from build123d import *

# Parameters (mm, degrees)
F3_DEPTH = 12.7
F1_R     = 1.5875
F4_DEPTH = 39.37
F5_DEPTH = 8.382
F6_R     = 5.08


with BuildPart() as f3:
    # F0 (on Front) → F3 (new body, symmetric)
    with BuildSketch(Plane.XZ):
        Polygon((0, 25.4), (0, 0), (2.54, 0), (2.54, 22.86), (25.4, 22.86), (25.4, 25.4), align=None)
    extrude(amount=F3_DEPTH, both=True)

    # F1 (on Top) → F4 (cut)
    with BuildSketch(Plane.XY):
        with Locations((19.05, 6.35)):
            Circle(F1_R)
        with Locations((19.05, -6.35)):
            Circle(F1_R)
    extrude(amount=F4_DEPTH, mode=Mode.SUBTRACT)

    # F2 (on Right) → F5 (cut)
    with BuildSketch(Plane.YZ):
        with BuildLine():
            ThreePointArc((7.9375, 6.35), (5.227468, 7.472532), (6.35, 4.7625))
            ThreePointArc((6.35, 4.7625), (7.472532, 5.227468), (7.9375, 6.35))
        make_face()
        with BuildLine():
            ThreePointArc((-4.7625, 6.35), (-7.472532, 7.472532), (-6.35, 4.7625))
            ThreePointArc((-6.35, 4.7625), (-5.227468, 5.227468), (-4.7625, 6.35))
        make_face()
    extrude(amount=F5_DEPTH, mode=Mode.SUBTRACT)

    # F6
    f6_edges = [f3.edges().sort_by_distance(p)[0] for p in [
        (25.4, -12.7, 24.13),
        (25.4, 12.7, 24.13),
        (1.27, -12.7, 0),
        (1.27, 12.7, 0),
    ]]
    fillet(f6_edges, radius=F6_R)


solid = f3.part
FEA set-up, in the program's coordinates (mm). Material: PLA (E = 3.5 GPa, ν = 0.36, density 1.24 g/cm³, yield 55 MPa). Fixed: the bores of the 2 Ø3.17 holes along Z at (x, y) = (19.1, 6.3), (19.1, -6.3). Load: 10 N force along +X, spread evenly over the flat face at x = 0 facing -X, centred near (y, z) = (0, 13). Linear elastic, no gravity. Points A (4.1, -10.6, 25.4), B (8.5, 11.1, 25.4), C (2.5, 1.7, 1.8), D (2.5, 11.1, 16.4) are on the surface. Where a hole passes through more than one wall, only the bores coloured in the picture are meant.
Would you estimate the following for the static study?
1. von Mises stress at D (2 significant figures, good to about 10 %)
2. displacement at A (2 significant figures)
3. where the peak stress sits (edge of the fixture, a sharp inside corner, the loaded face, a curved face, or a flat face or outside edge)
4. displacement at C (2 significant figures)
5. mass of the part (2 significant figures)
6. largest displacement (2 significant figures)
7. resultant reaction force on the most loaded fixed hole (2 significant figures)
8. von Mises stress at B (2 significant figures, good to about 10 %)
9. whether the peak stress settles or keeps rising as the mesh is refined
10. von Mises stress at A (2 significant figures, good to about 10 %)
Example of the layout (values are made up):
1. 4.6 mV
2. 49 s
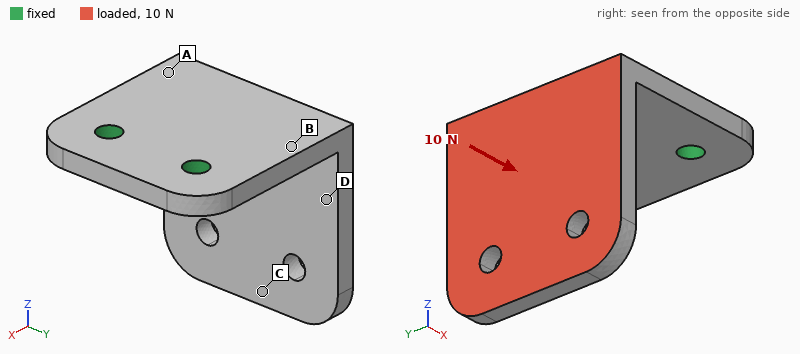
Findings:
1. 1.7 MPa
2. 0.091 mm
3. edge of the fixture
4. 0.43 mm
5. 3.7 g
6. 0.48 mm
7. 5.1 N
8. 4.0 MPa
9. keeps rising
10. 3.4 MPa
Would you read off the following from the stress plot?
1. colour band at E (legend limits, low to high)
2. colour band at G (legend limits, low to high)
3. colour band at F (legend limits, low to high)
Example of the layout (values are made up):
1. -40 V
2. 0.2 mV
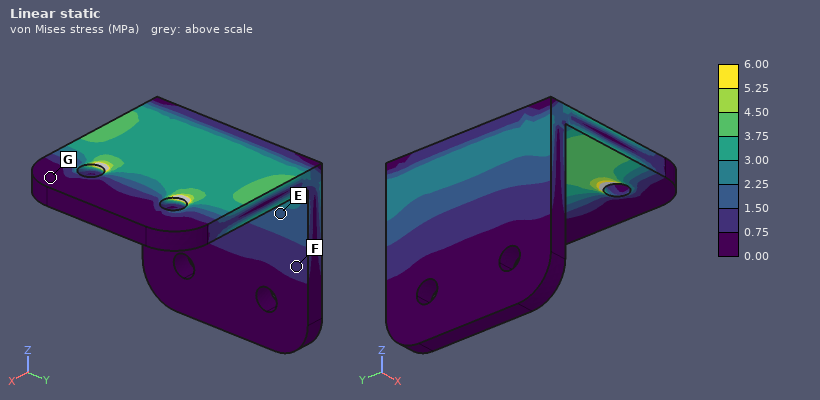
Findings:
1. 1.50 to 2.25 MPa
2. 0.00 to 0.75 MPa
3. 0.75 to 1.50 MPa
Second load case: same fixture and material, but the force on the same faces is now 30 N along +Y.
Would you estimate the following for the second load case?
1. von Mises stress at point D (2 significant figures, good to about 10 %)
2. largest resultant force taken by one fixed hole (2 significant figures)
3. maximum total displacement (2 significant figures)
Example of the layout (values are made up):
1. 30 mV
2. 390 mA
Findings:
1. 2.6 MPa
2. 45 N
3. 0.47 mm
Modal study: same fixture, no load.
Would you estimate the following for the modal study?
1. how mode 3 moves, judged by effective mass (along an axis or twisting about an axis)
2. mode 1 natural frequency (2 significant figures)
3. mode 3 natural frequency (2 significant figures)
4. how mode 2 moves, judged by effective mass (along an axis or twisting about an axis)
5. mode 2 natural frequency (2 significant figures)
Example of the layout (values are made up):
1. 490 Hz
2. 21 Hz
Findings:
1. along Z
2. 570 Hz
3. 1600 Hz
4. along Y
5. 990 Hz
